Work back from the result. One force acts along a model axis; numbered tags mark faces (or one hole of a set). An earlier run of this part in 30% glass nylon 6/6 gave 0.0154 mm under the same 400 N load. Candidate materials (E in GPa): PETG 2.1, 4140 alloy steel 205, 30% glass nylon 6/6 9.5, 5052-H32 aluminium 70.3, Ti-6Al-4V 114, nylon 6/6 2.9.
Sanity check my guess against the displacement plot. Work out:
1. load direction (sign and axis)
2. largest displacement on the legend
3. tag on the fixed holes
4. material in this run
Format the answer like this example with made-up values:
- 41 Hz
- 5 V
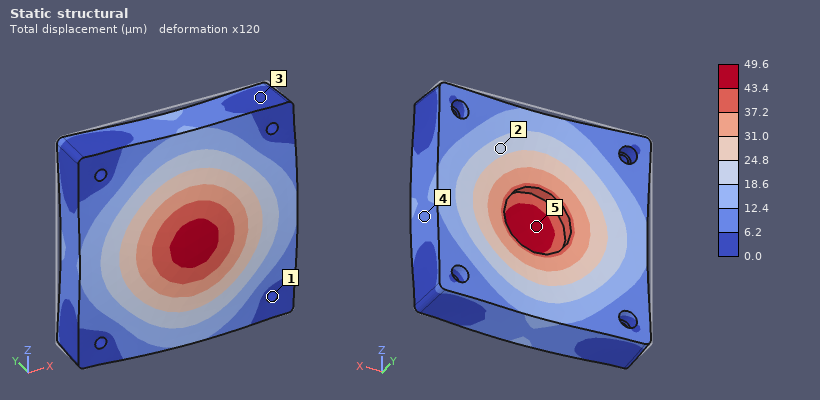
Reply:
- -Y
- 49.6 µm
- 1
- nylon 6/6
